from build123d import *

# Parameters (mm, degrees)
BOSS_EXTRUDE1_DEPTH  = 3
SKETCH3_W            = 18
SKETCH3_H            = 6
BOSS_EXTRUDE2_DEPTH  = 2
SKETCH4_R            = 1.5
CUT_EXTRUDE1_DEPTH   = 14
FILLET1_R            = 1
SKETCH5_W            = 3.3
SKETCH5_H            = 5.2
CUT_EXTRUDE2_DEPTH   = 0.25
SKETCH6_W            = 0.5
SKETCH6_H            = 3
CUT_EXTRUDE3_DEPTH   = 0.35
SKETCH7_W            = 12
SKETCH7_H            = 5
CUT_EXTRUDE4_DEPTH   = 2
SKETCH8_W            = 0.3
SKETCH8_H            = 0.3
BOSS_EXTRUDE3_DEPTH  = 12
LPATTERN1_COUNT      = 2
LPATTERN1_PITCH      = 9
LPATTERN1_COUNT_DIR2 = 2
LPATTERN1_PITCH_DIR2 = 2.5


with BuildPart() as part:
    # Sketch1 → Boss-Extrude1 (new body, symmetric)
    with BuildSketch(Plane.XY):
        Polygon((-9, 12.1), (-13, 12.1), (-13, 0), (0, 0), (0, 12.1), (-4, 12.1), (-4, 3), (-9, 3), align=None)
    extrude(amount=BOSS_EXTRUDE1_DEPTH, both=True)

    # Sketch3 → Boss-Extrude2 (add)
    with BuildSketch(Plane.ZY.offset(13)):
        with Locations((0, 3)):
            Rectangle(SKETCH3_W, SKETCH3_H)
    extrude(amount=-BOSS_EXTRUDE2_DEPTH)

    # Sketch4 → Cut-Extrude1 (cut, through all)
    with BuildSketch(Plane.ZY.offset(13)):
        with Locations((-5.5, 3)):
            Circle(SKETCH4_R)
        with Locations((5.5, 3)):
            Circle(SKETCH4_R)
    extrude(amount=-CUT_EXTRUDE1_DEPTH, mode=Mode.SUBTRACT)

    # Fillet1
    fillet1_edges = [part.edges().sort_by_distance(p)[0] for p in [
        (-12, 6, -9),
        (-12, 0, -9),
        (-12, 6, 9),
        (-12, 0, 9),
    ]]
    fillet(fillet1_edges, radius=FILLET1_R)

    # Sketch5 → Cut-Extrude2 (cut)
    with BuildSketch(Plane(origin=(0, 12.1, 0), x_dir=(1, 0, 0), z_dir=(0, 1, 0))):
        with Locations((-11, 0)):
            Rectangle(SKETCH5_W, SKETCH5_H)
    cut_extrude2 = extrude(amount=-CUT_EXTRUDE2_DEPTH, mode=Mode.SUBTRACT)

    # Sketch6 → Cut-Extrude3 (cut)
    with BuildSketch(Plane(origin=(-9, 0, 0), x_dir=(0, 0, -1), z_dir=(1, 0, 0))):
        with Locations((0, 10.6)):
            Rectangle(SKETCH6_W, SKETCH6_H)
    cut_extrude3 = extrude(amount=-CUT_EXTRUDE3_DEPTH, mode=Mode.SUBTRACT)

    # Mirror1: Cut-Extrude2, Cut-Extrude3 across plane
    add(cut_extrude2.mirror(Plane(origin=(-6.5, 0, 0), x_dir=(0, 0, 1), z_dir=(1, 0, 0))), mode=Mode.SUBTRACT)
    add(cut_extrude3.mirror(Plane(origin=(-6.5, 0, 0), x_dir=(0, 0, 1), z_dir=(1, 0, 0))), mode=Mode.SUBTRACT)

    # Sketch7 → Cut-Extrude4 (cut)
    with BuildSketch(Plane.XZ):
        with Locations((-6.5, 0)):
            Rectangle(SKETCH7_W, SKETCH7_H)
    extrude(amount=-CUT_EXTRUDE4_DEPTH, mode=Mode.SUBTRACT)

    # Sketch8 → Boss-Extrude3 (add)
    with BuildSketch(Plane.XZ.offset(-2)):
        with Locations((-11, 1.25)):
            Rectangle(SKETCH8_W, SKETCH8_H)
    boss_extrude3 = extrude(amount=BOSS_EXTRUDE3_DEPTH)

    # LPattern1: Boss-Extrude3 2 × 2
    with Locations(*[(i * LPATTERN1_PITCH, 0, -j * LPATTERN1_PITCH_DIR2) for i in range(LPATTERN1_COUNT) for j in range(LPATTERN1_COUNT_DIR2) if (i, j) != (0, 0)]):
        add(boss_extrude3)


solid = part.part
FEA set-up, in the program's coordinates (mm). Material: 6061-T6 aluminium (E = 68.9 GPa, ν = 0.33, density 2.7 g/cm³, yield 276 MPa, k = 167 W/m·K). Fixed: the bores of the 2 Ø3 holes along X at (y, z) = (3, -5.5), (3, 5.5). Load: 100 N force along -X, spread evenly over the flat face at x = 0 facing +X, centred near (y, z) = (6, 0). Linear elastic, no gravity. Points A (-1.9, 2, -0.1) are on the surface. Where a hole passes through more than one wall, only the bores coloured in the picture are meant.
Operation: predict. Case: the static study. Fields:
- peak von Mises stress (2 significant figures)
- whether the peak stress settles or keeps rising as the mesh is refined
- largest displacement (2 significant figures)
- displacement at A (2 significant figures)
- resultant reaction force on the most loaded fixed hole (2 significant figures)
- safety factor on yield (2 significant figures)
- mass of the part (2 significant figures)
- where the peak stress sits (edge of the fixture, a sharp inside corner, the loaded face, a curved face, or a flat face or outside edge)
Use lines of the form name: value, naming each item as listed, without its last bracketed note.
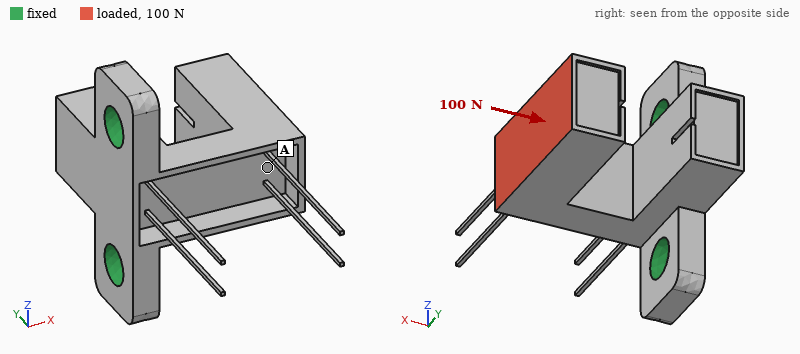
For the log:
peak von Mises stress: 180 MPa
whether the peak stress settles or keeps rising as the mesh is refined: settles
largest displacement: 0.15 mm
displacement at A: 0.053 mm
resultant reaction force on the most loaded fixed hole: 56 N
safety factor on yield: 1.6
mass of the part: 1.8 g
where the peak stress sits: a flat face or outside edge
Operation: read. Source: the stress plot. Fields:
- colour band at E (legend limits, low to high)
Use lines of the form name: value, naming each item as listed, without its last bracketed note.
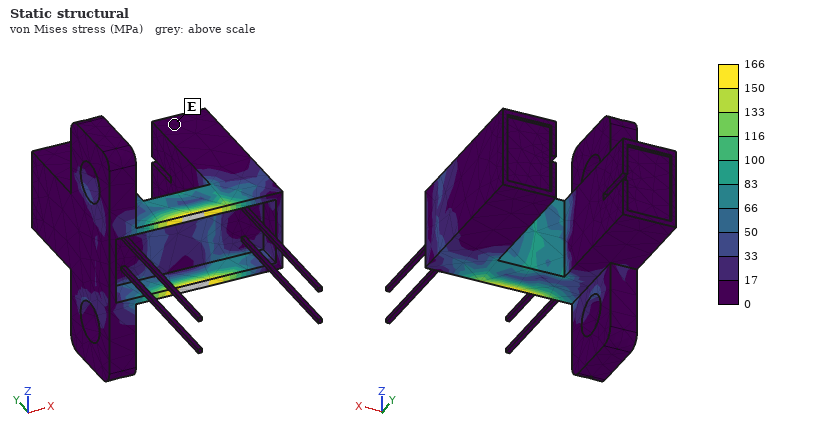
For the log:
colour band at E: 0 to 17 MPa
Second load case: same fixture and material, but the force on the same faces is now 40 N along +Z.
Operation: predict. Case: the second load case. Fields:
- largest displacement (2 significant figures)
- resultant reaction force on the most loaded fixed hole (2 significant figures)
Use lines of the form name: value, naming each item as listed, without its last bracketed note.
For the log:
largest displacement: 53 µm
resultant reaction force on the most loaded fixed hole: 74 N
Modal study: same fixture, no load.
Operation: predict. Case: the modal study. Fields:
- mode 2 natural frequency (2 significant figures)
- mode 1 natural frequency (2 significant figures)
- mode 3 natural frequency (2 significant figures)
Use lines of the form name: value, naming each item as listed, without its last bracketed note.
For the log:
mode 2 natural frequency: 1700 Hz
mode 1 natural frequency: 1700 Hz
mode 3 natural frequency: 1700 Hz
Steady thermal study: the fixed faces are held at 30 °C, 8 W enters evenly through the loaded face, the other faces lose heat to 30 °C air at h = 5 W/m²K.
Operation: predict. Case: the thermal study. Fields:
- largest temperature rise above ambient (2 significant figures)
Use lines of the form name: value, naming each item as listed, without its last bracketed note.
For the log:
largest temperature rise above ambient: 57 K
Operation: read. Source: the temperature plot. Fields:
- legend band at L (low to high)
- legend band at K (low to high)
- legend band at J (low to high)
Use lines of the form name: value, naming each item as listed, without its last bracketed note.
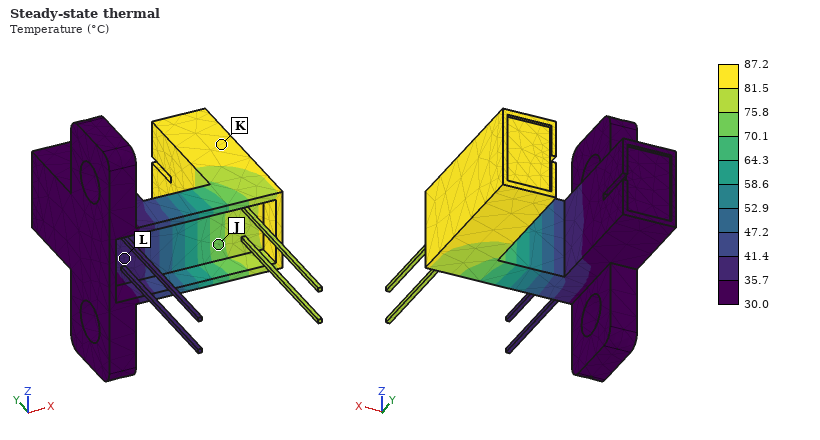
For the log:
legend band at L: 35.7 to 41.4 °C
legend band at K: 81.5 to 87.2 °C
legend band at J: 70.1 to 75.8 °C
